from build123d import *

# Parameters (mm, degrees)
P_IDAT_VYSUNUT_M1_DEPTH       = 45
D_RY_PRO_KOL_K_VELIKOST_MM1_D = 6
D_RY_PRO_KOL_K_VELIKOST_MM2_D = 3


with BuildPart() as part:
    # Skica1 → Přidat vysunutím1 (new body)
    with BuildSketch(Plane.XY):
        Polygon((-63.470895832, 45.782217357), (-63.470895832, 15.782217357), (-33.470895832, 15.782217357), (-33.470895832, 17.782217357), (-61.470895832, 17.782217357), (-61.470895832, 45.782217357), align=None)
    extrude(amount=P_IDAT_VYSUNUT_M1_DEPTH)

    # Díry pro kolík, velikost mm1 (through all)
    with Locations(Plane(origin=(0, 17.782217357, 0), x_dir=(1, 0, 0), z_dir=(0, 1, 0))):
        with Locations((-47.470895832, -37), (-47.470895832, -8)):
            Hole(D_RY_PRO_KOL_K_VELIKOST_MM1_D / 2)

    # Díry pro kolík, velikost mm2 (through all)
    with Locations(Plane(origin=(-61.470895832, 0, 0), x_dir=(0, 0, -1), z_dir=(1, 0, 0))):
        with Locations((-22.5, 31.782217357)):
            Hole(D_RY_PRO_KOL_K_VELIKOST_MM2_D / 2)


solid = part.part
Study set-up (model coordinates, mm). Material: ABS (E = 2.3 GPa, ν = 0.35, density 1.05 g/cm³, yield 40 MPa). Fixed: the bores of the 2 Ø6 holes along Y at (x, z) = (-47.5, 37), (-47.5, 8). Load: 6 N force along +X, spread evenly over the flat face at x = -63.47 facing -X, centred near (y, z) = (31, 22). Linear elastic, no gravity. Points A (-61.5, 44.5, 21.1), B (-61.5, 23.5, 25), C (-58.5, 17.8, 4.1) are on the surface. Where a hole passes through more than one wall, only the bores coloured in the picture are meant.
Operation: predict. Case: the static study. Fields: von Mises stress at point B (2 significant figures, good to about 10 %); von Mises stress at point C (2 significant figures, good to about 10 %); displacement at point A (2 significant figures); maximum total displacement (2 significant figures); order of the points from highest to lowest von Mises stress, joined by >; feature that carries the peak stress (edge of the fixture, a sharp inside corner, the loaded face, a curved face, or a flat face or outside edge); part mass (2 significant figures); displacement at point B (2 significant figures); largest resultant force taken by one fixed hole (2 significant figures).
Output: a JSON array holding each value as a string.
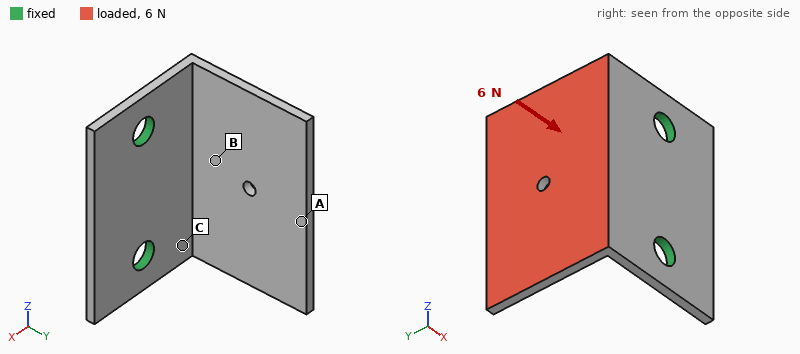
["1.5 MPa", "2.5 MPa", "0.62 mm", "0.66 mm", "C > B > A", "a flat face or outside edge", "5.3 g", "0.14 mm", "3.1 N"]
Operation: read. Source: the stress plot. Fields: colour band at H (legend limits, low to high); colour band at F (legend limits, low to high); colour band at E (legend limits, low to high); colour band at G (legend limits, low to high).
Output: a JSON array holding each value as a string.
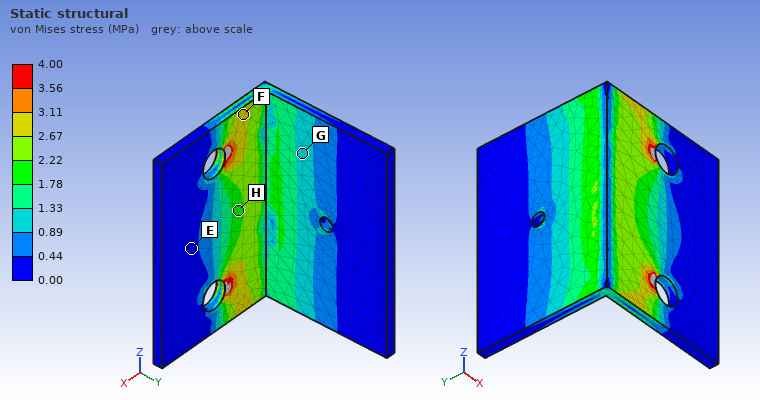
["1.78 to 2.22 MPa", "2.67 to 3.11 MPa", "0.00 to 0.44 MPa", "0.89 to 1.33 MPa"]
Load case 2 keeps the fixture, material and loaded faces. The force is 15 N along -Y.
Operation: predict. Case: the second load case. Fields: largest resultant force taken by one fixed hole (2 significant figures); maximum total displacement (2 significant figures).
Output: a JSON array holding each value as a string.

["7.5 N", "0.70 mm"]
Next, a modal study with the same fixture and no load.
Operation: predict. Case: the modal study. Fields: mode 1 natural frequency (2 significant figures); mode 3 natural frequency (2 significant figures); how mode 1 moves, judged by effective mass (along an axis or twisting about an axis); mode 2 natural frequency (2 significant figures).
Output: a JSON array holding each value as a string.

["340 Hz", "1100 Hz", "along X", "700 Hz"]
